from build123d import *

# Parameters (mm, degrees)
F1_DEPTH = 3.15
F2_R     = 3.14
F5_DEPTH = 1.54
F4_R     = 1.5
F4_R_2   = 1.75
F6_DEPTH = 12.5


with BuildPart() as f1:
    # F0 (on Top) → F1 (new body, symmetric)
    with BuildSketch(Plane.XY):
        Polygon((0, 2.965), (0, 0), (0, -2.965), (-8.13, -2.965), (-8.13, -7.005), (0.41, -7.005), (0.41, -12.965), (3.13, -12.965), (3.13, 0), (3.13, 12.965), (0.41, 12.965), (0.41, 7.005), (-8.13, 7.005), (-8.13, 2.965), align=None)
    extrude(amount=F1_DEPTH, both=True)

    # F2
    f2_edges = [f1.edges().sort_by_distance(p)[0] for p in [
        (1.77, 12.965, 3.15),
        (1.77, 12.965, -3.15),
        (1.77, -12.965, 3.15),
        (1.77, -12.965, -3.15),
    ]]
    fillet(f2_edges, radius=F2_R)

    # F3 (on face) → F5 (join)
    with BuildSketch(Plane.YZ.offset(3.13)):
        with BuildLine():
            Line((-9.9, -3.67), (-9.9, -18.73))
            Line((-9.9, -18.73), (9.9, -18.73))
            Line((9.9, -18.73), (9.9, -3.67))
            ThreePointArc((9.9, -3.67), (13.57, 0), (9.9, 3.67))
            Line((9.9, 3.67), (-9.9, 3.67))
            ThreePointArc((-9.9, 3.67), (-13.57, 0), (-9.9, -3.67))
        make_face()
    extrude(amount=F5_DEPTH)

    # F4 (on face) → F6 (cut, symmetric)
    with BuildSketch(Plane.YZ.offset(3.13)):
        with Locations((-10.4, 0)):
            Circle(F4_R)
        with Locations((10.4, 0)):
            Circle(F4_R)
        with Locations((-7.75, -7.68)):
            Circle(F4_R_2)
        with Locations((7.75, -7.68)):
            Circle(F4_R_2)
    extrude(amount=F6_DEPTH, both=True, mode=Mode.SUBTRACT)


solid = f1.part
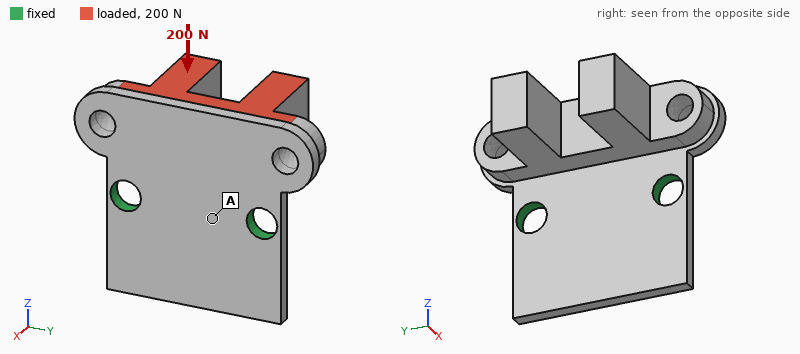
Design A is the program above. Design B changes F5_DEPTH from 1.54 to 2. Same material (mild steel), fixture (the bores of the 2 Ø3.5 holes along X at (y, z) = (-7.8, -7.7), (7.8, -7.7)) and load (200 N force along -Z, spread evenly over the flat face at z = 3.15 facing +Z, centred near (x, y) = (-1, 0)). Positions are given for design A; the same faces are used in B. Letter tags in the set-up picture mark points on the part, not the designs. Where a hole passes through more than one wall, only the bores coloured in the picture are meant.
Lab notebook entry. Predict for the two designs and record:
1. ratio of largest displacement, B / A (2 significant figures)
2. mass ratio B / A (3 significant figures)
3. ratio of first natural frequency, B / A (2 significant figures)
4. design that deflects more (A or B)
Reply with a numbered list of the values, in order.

1. 0.53
2. 1.14
3. 1.4
4. A
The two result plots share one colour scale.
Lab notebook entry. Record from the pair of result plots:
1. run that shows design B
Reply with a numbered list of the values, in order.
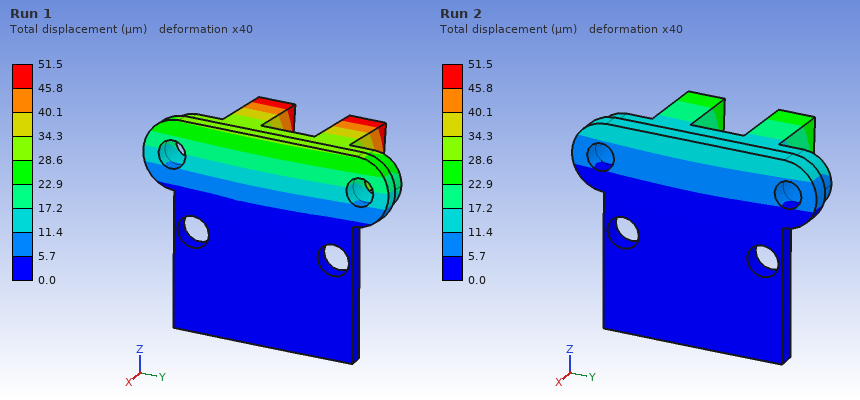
1. Run 2
